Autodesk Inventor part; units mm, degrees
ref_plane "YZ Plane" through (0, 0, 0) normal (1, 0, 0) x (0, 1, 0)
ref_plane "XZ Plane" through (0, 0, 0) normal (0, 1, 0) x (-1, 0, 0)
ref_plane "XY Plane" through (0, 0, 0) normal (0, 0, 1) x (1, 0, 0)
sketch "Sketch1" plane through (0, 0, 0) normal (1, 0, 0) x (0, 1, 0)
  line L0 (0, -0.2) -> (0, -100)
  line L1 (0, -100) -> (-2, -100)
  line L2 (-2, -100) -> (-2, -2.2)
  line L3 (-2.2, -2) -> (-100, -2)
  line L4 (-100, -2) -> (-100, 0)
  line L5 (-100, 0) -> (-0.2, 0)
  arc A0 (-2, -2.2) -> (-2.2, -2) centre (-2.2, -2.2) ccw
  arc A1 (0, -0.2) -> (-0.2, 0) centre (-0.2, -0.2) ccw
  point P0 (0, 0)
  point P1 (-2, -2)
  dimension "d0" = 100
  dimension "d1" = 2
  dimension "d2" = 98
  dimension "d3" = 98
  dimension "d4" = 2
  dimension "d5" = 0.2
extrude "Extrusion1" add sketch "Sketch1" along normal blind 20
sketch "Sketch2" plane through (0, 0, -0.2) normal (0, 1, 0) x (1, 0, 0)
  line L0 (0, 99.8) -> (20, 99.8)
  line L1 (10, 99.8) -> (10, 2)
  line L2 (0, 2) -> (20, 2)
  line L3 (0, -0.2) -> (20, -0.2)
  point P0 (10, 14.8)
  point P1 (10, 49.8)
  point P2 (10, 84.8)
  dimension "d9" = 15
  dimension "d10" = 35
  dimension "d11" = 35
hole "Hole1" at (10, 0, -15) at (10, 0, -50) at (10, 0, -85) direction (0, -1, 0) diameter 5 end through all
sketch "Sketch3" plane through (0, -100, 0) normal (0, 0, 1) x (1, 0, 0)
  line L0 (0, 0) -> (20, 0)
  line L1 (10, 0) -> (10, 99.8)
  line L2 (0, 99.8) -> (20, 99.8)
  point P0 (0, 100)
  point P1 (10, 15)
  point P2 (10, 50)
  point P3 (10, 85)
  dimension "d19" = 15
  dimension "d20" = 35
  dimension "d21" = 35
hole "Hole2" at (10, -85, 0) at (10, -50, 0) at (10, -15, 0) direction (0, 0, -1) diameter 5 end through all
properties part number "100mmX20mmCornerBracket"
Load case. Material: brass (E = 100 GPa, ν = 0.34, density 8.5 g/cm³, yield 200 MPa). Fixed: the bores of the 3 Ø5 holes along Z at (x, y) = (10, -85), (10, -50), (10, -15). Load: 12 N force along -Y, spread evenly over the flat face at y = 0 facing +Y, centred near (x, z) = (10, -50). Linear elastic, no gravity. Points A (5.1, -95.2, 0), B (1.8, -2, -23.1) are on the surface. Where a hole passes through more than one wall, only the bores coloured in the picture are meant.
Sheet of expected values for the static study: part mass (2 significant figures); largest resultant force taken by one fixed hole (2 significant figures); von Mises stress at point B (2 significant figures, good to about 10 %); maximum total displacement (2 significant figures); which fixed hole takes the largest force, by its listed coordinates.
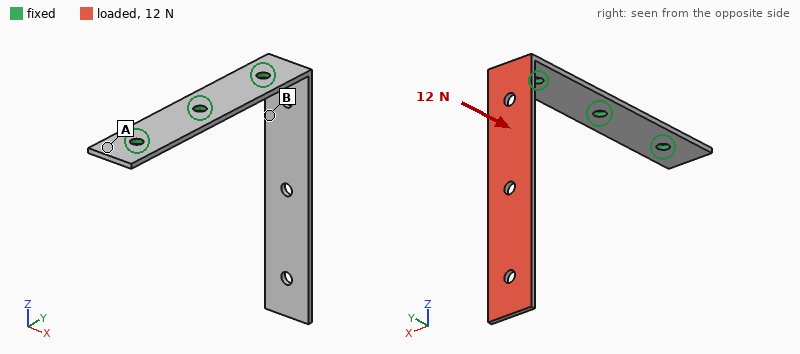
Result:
65 g
12 N
28 MPa
1.6 mm
(10, -15)
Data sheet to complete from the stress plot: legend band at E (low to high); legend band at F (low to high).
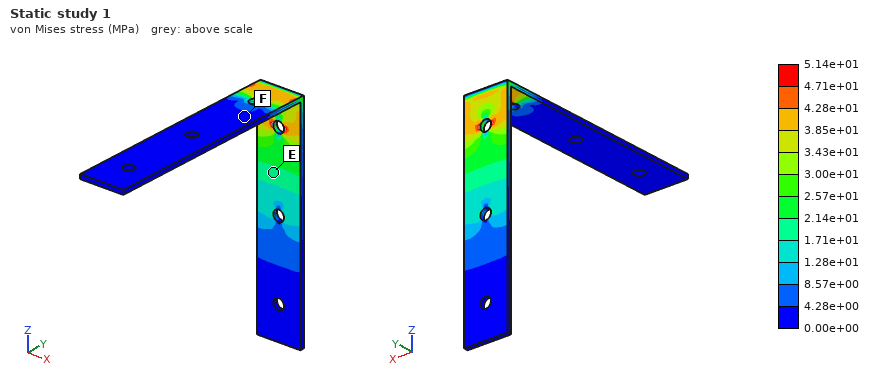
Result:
1.71e+01 to 2.14e+01 MPa
0.00e+00 to 4.28e+00 MPa
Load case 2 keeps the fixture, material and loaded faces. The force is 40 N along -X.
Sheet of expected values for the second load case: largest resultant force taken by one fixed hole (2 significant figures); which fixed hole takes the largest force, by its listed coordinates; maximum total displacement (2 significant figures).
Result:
51 N
(10, -15)
0.99 mm
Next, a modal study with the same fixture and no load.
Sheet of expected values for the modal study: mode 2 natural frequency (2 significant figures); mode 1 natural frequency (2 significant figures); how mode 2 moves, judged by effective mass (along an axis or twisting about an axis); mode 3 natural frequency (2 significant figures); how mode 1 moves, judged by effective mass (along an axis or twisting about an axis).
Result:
210 Hz
94 Hz
along X
600 Hz
along Y
